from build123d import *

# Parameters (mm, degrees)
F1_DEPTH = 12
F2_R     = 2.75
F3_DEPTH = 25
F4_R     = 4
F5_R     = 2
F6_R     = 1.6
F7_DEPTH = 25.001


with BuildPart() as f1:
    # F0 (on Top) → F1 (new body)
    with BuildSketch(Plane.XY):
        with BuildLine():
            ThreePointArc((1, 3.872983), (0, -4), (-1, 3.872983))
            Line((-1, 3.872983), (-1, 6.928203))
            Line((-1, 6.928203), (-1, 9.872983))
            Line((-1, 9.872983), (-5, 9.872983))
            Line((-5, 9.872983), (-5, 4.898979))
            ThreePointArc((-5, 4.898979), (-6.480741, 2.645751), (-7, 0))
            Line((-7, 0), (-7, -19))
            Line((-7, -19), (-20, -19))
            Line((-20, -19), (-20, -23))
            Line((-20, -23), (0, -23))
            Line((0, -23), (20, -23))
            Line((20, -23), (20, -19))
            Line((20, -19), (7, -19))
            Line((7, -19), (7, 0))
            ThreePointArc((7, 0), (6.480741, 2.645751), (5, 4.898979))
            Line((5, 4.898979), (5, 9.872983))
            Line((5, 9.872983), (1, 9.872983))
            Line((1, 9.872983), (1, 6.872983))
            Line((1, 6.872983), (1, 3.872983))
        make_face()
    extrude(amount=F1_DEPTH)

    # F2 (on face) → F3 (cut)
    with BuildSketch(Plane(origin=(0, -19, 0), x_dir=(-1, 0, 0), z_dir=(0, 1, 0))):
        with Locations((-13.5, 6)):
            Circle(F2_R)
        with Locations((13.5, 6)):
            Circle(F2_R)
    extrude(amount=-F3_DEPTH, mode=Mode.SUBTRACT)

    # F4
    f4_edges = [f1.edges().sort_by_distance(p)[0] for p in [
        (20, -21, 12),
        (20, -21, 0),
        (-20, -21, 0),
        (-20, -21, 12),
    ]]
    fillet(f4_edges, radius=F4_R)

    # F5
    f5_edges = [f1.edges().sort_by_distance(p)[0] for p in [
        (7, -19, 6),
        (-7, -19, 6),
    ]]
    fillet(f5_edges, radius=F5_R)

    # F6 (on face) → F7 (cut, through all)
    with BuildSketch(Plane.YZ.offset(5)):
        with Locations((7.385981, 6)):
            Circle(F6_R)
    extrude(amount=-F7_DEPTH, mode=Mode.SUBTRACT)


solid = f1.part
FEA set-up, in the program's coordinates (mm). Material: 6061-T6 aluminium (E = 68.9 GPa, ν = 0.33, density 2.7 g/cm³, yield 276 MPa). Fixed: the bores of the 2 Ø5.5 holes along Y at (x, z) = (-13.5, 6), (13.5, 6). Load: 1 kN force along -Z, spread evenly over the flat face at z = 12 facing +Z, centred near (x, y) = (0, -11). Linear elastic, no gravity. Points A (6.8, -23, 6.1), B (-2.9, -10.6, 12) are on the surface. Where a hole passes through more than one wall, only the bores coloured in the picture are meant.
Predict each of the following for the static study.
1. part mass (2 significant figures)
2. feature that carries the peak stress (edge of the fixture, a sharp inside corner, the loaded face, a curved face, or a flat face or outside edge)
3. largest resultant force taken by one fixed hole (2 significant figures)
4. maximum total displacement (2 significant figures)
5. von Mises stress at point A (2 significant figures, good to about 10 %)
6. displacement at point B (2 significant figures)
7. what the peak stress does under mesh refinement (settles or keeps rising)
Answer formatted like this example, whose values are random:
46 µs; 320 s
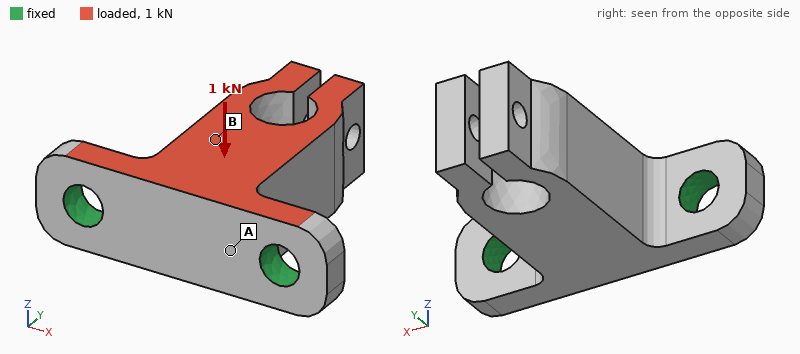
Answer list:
15 g; edge of the fixture; 500 N; 0.13 mm; 44 MPa; 0.049 mm; keeps rising
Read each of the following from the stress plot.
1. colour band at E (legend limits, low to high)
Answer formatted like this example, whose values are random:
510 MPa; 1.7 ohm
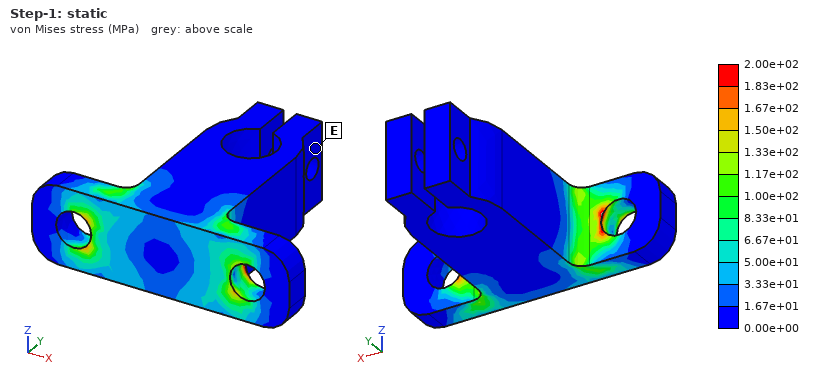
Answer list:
0.00e+00 to 1.67e+01 MPa
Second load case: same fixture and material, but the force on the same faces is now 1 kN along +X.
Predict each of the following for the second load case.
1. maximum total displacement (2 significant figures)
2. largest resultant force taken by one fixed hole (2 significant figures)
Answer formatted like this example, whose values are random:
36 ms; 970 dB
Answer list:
55 µm; 760 N
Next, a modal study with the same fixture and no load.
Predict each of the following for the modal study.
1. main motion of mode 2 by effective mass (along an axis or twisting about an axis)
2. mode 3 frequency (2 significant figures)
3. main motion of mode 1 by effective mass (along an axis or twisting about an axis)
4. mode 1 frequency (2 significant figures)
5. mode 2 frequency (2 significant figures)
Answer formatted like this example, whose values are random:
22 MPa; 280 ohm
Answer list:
along X; 12 kHz; along Z; 4800 Hz; 8600 Hz
